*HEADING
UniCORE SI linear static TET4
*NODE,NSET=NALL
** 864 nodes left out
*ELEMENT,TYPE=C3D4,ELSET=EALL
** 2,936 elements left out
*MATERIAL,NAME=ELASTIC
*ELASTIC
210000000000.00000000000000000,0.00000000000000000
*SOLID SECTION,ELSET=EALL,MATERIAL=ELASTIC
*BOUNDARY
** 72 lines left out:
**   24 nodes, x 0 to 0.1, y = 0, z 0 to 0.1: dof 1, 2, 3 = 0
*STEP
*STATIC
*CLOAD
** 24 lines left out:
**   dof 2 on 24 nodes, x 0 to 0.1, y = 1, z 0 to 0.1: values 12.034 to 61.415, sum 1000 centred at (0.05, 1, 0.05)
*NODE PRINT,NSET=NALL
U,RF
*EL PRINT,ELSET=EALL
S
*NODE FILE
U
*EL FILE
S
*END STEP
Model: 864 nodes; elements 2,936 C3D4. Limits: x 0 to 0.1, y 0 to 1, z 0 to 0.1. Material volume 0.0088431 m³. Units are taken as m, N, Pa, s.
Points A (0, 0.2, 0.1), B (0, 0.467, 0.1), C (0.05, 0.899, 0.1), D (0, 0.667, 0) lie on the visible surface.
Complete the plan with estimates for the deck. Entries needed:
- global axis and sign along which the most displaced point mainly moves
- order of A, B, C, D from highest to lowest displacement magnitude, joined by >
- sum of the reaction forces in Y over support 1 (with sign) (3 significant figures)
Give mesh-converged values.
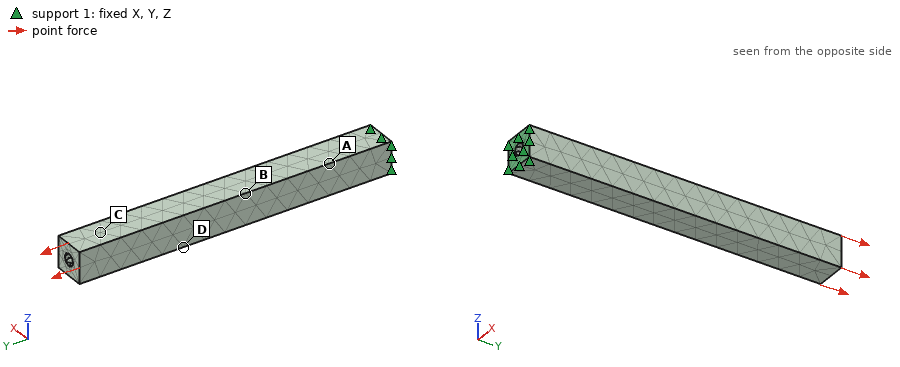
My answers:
+Y
C > D > B > A
-1000 N
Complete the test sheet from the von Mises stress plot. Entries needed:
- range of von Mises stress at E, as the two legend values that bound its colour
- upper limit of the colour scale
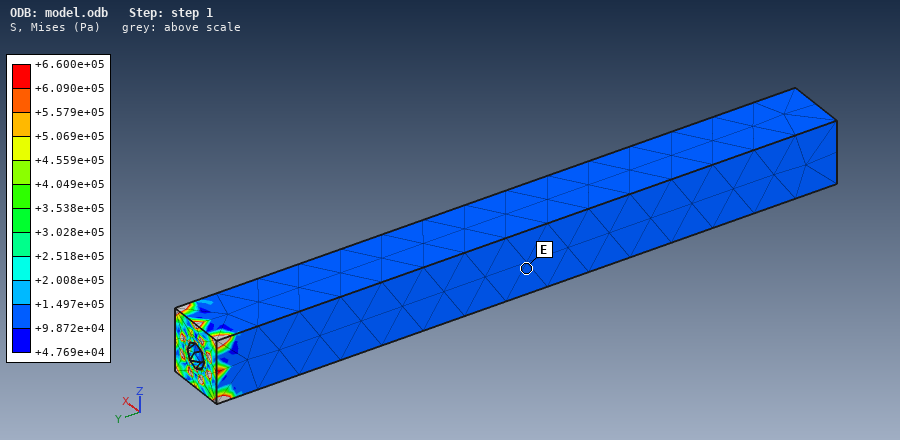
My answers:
+9.872e+04 to +1.497e+05 Pa
+6.600e+05 Pa
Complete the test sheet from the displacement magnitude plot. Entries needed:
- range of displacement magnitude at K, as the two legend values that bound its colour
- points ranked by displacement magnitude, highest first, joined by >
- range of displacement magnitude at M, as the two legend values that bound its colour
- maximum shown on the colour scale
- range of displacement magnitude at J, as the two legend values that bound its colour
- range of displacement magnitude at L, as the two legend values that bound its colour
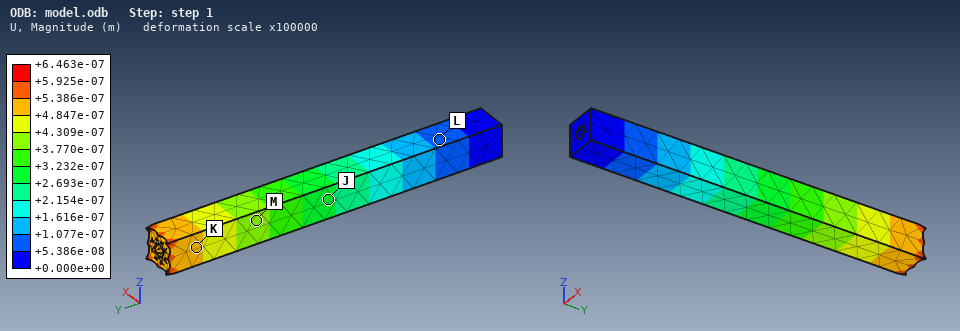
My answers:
+4.847e-07 to +5.386e-07 m
K > M > J > L
+3.770e-07 to +4.309e-07 m
+6.463e-07 m
+2.693e-07 to +3.232e-07 m
+5.386e-08 to +1.077e-07 m
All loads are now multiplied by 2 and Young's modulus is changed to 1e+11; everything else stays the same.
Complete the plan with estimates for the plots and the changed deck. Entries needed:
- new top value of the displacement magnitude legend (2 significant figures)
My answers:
2.7e-06 m
